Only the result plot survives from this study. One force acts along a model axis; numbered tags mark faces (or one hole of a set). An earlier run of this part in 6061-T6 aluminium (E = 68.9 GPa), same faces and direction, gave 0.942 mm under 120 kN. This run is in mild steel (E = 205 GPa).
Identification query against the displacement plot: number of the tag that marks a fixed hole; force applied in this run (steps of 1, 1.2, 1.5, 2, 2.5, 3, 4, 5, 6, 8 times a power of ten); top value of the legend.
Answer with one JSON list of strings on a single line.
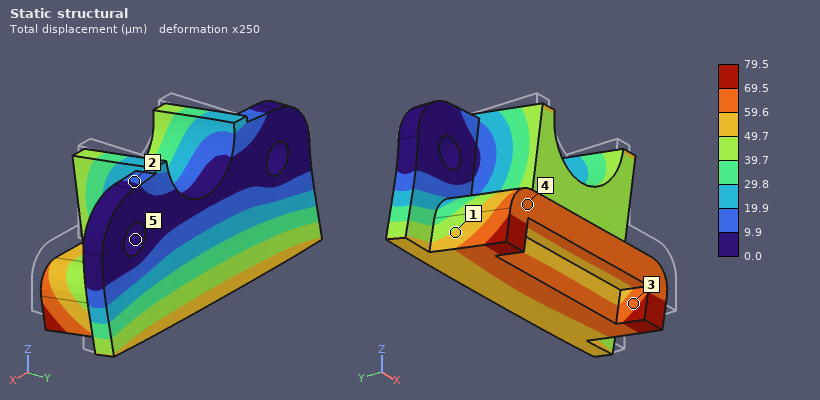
["5", "30 kN", "79.5 µm"]
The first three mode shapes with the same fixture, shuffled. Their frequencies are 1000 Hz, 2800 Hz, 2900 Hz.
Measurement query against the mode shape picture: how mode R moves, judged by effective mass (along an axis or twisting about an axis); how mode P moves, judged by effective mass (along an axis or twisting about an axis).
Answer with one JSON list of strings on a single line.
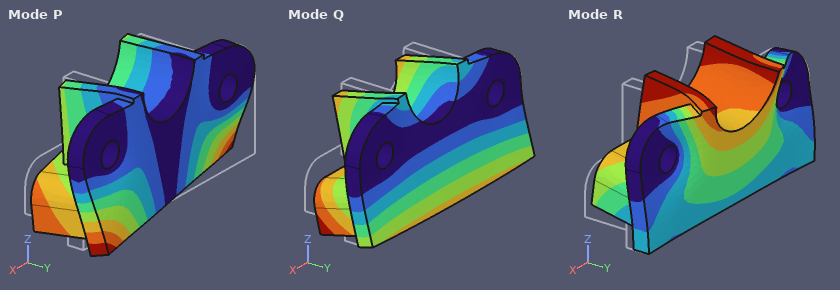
["along Y", "along X"]
